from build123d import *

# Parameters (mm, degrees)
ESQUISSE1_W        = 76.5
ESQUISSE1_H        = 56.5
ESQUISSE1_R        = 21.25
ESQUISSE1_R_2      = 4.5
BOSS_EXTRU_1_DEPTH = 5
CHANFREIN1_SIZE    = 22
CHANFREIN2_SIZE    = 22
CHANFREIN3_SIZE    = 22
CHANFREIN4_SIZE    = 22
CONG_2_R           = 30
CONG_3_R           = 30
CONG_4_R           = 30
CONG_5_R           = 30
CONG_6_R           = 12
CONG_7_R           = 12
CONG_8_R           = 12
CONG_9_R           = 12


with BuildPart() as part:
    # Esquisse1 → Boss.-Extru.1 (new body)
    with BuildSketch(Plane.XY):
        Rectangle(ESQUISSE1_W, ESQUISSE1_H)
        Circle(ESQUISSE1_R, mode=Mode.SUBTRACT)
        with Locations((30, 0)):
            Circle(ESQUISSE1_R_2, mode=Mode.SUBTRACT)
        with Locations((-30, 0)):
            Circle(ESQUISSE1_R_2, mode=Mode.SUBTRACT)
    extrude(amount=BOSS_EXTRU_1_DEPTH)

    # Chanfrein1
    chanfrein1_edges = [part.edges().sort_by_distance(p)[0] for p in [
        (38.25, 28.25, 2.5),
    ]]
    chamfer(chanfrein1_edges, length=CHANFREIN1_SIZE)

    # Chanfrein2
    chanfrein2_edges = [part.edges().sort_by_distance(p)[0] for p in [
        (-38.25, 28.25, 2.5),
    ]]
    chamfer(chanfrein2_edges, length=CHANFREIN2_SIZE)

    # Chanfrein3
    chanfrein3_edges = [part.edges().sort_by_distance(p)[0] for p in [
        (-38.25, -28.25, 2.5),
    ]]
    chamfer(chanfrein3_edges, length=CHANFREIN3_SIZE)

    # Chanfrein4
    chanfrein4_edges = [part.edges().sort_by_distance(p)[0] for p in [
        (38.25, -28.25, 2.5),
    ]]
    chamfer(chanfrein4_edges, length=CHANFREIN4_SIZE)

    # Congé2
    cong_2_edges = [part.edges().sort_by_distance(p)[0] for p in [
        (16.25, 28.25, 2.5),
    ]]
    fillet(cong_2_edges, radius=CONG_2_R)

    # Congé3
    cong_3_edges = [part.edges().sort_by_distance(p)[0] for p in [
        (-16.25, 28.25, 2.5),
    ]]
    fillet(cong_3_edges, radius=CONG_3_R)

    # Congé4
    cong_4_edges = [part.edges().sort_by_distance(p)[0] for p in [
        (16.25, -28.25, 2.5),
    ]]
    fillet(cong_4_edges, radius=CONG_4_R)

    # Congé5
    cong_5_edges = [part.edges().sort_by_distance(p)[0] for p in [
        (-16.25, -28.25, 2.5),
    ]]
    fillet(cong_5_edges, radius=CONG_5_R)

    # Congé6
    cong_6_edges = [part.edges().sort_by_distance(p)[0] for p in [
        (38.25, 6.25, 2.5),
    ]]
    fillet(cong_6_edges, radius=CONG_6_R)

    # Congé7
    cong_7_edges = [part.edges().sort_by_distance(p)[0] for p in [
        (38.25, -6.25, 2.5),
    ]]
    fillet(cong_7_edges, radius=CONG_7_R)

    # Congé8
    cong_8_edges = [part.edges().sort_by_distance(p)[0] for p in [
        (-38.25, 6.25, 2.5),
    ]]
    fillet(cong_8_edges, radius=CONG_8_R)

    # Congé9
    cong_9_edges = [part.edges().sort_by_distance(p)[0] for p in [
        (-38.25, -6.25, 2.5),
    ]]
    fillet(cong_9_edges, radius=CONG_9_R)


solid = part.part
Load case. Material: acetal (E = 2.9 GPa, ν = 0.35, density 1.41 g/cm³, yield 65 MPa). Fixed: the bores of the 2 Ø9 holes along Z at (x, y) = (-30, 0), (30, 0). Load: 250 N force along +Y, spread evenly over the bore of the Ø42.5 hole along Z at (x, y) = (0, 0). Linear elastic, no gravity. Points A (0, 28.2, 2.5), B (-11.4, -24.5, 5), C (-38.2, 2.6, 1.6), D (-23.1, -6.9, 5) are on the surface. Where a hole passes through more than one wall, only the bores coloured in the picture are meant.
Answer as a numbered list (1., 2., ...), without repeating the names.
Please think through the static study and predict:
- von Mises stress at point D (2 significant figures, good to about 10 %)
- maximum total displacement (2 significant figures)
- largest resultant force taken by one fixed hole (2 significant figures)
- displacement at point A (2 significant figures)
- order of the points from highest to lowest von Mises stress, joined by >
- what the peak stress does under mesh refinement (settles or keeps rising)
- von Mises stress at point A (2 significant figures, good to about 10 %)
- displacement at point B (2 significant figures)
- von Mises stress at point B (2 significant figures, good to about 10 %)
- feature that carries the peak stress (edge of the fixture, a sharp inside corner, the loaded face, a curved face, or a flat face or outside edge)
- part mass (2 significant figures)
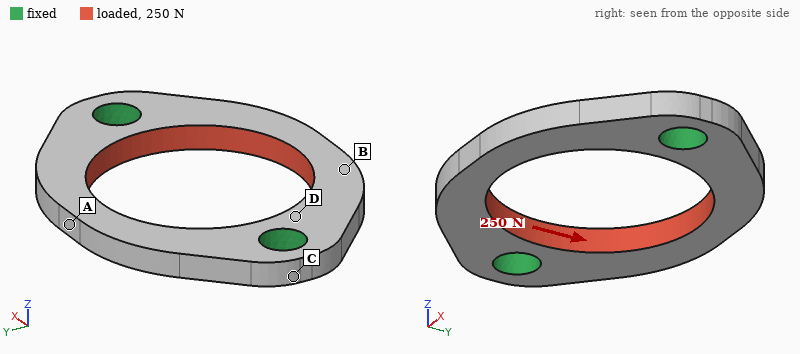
1. 1.6 MPa
2. 26 µm
3. 130 N
4. 24 µm
5. A > D > B > C
6. keeps rising
7. 2.3 MPa
8. 18 µm
9. 1.1 MPa
10. edge of the fixture
11. 12 g
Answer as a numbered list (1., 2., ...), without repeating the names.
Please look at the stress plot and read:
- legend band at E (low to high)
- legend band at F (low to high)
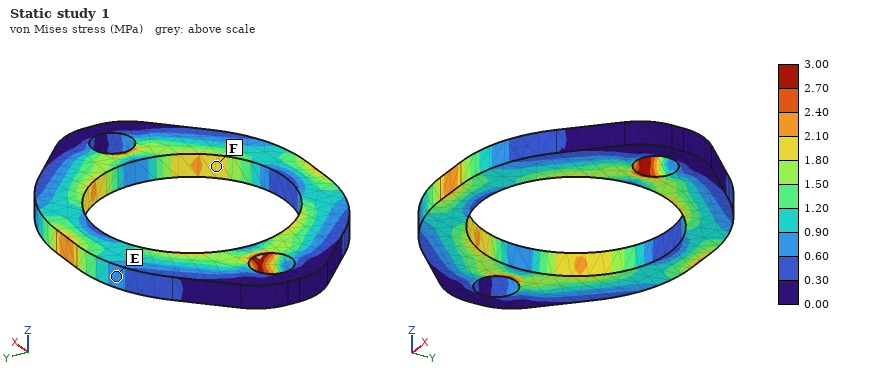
1. 0.60 to 0.90 MPa
2. 1.80 to 2.10 MPa
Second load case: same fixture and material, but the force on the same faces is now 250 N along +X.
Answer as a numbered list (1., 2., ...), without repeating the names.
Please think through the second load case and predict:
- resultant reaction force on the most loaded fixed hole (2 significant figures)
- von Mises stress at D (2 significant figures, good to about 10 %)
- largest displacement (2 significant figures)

1. 130 N
2. 1.4 MPa
3. 29 µm
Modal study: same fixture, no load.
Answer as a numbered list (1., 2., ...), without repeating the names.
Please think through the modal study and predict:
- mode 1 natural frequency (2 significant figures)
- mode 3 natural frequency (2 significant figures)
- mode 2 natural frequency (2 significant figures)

1. 1200 Hz
2. 3000 Hz
3. 1300 Hz
